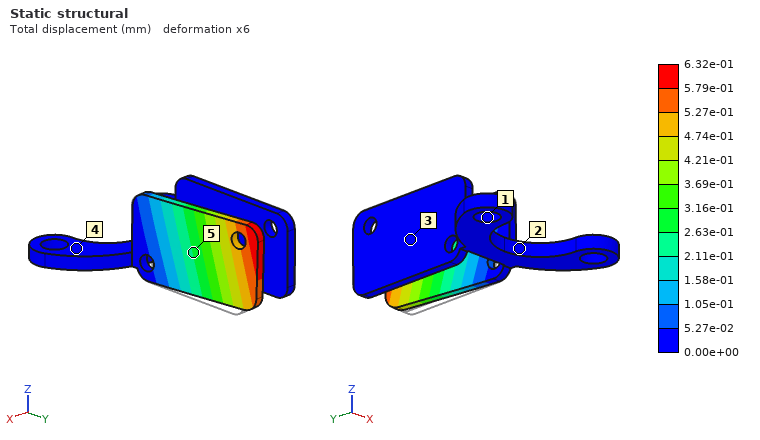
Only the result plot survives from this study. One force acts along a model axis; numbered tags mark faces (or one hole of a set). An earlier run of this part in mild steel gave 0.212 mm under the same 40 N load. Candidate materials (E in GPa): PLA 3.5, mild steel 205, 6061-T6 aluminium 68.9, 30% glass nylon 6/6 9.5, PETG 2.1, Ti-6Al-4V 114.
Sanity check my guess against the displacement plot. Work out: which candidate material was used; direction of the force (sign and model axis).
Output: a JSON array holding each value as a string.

["6061-T6 aluminium", "-X"]
